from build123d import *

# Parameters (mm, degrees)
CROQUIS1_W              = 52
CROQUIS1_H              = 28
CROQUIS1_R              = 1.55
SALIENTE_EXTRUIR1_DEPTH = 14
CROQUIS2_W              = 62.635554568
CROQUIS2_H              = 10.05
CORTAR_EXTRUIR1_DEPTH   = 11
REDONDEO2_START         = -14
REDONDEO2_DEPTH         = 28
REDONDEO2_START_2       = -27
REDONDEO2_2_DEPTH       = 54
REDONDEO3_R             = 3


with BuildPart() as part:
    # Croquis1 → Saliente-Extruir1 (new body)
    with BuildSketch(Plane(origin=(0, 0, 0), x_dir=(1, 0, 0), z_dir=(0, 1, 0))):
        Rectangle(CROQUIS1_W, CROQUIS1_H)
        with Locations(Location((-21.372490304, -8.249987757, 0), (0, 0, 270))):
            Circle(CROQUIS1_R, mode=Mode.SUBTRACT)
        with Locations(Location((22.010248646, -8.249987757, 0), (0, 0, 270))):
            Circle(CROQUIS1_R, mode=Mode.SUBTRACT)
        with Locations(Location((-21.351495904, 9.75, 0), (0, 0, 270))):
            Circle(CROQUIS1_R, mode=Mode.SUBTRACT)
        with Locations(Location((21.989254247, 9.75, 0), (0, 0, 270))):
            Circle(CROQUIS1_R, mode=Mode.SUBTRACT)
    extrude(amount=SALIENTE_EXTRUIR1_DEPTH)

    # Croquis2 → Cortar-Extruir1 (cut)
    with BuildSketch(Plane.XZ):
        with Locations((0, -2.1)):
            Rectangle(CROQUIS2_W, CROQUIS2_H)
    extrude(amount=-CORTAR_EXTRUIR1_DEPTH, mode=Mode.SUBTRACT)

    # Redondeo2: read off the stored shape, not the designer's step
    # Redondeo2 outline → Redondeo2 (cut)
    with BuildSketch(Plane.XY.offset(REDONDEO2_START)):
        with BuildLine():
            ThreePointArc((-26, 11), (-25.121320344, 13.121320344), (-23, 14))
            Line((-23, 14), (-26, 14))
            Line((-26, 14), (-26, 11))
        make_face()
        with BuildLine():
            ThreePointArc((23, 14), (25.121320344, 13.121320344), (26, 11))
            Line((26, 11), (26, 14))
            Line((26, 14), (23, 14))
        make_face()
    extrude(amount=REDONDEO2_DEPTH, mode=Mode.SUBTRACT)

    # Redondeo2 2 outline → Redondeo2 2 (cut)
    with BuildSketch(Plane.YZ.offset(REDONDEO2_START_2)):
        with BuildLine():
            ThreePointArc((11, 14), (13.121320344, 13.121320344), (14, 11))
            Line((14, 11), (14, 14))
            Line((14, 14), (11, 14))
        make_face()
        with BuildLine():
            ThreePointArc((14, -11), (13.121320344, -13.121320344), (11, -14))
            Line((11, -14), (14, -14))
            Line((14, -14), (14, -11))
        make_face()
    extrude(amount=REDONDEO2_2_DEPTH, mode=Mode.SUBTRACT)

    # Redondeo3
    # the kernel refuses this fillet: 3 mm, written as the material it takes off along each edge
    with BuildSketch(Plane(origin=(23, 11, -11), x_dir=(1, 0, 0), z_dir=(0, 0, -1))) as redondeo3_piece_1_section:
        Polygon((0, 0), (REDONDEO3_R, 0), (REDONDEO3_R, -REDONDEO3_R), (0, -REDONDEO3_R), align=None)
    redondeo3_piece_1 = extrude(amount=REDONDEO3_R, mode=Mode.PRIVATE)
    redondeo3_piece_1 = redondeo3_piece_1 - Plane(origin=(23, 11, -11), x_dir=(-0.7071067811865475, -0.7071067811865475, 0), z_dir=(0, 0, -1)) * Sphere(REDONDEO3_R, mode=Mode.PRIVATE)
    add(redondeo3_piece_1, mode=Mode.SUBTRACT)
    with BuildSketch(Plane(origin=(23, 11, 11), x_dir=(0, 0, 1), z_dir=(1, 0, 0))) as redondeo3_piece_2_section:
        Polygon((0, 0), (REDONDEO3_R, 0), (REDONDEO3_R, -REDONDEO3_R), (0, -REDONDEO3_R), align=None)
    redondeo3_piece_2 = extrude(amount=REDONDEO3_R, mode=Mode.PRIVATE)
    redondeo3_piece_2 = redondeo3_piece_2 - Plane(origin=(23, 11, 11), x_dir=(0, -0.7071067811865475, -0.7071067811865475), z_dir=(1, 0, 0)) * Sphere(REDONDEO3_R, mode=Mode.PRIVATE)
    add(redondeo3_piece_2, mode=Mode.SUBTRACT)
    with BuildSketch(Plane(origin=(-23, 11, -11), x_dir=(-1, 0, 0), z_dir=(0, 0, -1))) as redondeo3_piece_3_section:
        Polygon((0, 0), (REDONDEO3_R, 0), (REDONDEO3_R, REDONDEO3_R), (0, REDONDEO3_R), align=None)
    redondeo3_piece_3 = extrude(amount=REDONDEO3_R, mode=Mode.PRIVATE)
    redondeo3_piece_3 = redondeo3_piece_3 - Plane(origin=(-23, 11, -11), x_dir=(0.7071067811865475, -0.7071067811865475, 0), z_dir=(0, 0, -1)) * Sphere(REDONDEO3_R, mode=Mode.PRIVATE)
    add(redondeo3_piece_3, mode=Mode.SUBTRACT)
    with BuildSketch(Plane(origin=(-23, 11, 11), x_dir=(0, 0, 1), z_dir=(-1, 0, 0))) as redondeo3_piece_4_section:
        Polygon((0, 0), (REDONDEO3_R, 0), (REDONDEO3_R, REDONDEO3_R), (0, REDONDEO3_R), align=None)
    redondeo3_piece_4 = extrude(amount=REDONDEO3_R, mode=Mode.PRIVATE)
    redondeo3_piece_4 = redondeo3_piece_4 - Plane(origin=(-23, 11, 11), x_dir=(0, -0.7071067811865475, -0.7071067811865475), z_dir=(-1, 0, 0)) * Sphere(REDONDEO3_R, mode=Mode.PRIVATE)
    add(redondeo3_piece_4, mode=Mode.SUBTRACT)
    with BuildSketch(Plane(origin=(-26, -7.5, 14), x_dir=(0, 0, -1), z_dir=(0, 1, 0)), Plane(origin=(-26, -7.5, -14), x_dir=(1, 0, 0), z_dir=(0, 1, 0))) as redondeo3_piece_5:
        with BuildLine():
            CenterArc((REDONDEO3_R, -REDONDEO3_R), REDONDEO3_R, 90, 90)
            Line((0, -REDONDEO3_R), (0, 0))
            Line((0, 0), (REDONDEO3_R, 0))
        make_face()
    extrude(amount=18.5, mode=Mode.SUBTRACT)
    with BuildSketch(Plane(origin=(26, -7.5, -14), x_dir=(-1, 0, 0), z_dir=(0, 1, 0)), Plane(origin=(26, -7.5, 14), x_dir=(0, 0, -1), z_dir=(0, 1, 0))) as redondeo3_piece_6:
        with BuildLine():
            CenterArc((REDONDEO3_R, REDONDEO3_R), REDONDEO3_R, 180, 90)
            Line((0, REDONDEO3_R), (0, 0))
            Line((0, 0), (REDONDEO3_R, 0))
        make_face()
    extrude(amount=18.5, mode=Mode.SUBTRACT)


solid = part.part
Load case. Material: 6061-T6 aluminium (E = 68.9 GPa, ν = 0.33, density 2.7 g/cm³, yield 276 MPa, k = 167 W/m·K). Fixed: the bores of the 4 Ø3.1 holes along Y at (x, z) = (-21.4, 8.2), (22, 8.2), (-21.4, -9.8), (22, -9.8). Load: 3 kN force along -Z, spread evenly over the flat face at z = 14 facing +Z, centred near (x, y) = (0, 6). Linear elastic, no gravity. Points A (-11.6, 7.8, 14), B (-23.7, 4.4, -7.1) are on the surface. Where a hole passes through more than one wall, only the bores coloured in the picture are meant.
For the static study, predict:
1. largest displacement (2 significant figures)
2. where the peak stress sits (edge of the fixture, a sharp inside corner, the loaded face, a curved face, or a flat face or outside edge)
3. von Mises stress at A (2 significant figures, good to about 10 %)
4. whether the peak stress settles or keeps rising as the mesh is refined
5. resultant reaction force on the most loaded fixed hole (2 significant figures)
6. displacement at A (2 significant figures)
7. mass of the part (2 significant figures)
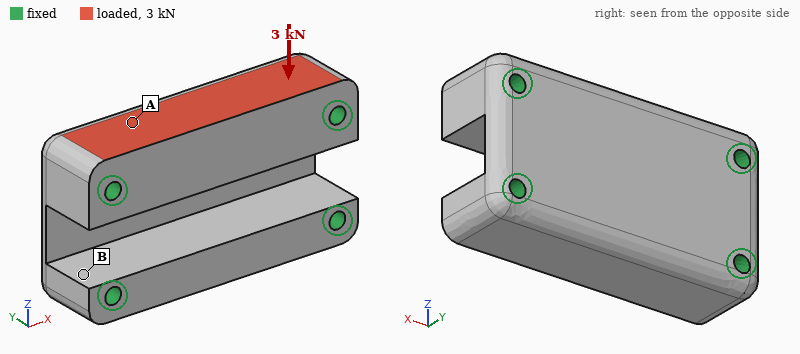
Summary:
13 µm
edge of the fixture
14 MPa
keeps rising
1.3 kN
6.0 µm
37 g
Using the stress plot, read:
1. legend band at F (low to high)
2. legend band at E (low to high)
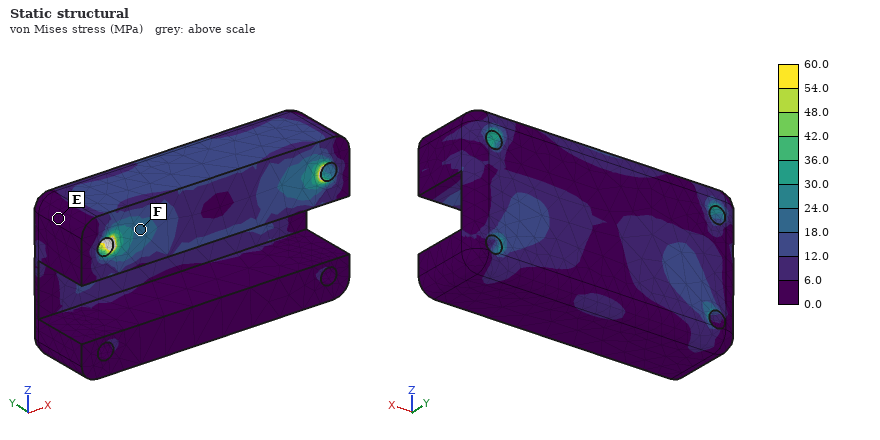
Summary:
18.0 to 24.0 MPa
0.0 to 6.0 MPa
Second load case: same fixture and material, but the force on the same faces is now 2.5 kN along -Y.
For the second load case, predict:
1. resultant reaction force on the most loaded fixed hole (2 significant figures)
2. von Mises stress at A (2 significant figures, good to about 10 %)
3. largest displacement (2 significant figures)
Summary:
1.3 kN
26 MPa
14 µm
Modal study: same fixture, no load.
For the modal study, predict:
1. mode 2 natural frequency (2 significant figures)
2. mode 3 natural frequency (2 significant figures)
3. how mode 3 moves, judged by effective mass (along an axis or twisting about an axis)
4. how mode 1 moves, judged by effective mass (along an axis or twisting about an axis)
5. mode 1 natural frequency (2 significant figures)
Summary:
23 kHz
25 kHz
along Y
along Z
21 kHz
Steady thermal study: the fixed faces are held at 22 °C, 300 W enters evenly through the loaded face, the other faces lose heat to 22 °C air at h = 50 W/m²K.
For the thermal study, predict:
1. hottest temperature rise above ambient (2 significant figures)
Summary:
66 K
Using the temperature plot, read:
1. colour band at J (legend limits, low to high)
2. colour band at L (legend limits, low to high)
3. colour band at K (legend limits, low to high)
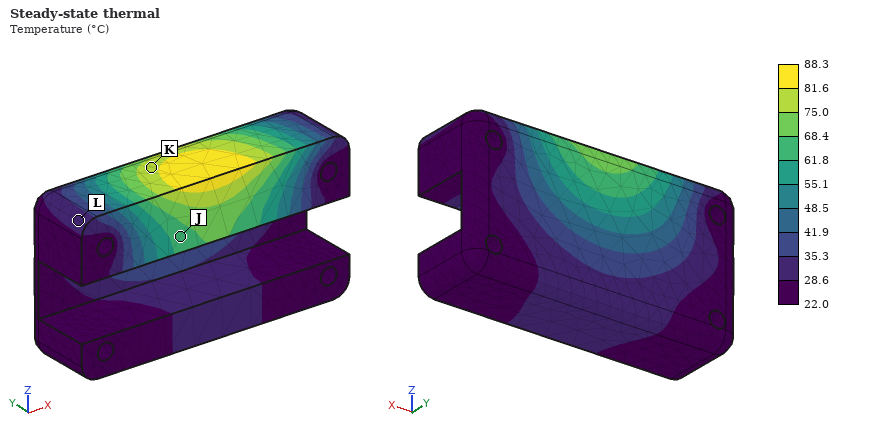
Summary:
61.8 to 68.4 °C
28.6 to 35.3 °C
75.0 to 81.6 °C
